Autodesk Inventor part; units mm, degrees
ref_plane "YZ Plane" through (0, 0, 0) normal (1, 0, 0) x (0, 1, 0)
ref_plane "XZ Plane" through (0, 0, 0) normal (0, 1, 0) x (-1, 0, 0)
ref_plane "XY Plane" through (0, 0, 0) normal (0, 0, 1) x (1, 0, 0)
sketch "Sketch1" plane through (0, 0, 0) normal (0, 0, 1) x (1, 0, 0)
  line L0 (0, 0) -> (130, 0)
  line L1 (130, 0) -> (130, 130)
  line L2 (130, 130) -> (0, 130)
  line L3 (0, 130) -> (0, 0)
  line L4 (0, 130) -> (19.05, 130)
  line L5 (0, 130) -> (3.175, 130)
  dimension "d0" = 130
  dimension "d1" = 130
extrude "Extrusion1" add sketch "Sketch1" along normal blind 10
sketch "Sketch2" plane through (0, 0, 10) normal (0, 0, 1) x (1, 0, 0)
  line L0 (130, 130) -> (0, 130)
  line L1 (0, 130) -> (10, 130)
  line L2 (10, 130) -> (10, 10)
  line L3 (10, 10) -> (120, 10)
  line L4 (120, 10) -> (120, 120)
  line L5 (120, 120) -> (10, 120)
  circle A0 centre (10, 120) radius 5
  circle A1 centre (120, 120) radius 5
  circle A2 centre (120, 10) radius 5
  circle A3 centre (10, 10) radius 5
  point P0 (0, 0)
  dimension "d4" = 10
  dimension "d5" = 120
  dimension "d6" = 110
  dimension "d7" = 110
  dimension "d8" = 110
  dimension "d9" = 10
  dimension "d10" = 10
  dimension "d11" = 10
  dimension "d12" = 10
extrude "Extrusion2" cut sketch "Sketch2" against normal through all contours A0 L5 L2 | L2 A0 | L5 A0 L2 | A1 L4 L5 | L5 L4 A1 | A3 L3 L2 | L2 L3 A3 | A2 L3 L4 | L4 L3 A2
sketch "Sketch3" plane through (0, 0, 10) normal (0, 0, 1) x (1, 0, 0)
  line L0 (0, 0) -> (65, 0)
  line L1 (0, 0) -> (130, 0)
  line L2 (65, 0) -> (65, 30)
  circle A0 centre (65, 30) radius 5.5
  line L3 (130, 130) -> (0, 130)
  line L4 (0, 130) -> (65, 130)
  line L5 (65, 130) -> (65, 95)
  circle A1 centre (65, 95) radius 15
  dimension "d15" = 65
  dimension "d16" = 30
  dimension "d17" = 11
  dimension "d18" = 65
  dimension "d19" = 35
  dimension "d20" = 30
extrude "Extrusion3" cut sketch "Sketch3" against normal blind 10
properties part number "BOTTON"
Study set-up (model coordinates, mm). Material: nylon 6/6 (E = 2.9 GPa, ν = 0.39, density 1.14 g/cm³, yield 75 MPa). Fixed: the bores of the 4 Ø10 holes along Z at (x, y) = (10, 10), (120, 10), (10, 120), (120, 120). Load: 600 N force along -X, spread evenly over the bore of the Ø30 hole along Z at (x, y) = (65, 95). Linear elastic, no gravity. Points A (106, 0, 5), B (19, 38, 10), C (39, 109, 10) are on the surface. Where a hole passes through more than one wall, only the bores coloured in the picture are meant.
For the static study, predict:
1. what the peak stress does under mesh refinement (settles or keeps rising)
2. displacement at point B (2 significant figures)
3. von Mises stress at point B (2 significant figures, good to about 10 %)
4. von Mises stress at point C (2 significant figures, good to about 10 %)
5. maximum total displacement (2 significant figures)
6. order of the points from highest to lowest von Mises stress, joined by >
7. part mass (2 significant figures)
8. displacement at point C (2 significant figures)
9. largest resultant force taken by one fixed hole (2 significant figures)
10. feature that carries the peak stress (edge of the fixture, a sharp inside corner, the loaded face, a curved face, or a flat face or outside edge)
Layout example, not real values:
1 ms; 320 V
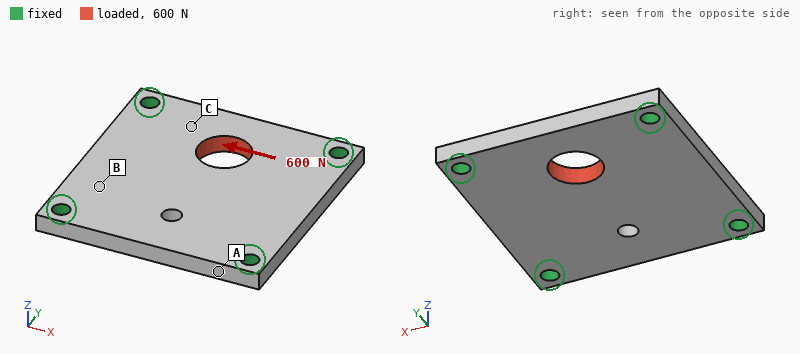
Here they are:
keeps rising; 5.7 µm; 0.31 MPa; 0.65 MPa; 16 µm; C > B > A; 180 g; 8.6 µm; 220 N; edge of the fixture
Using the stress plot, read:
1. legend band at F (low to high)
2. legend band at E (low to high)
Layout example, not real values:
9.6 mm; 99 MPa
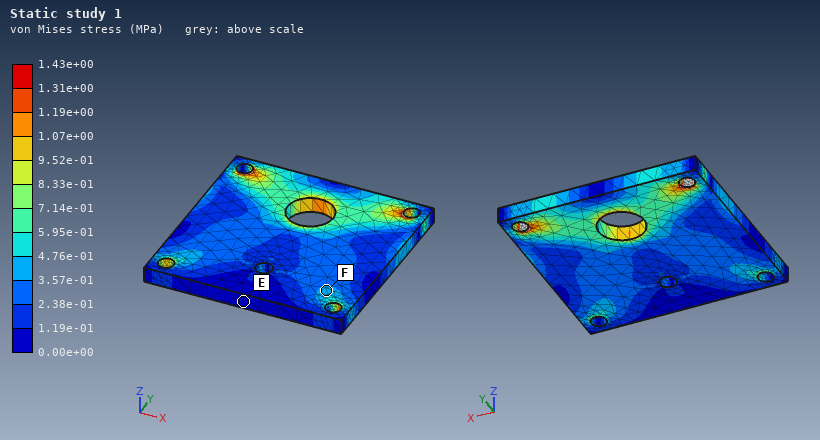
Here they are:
3.57e-01 to 4.76e-01 MPa; 0.00e+00 to 1.19e-01 MPa
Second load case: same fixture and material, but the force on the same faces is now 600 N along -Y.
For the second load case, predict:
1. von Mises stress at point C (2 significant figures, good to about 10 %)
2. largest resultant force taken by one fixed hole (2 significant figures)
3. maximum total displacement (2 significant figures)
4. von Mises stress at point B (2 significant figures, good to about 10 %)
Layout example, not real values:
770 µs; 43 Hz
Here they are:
0.56 MPa; 170 N; 28 µm; 0.43 MPa
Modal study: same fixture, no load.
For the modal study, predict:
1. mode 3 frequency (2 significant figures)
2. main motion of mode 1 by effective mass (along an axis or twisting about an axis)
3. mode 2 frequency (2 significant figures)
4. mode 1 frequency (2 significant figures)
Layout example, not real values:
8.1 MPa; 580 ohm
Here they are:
1500 Hz; along Z; 1500 Hz; 910 Hz
